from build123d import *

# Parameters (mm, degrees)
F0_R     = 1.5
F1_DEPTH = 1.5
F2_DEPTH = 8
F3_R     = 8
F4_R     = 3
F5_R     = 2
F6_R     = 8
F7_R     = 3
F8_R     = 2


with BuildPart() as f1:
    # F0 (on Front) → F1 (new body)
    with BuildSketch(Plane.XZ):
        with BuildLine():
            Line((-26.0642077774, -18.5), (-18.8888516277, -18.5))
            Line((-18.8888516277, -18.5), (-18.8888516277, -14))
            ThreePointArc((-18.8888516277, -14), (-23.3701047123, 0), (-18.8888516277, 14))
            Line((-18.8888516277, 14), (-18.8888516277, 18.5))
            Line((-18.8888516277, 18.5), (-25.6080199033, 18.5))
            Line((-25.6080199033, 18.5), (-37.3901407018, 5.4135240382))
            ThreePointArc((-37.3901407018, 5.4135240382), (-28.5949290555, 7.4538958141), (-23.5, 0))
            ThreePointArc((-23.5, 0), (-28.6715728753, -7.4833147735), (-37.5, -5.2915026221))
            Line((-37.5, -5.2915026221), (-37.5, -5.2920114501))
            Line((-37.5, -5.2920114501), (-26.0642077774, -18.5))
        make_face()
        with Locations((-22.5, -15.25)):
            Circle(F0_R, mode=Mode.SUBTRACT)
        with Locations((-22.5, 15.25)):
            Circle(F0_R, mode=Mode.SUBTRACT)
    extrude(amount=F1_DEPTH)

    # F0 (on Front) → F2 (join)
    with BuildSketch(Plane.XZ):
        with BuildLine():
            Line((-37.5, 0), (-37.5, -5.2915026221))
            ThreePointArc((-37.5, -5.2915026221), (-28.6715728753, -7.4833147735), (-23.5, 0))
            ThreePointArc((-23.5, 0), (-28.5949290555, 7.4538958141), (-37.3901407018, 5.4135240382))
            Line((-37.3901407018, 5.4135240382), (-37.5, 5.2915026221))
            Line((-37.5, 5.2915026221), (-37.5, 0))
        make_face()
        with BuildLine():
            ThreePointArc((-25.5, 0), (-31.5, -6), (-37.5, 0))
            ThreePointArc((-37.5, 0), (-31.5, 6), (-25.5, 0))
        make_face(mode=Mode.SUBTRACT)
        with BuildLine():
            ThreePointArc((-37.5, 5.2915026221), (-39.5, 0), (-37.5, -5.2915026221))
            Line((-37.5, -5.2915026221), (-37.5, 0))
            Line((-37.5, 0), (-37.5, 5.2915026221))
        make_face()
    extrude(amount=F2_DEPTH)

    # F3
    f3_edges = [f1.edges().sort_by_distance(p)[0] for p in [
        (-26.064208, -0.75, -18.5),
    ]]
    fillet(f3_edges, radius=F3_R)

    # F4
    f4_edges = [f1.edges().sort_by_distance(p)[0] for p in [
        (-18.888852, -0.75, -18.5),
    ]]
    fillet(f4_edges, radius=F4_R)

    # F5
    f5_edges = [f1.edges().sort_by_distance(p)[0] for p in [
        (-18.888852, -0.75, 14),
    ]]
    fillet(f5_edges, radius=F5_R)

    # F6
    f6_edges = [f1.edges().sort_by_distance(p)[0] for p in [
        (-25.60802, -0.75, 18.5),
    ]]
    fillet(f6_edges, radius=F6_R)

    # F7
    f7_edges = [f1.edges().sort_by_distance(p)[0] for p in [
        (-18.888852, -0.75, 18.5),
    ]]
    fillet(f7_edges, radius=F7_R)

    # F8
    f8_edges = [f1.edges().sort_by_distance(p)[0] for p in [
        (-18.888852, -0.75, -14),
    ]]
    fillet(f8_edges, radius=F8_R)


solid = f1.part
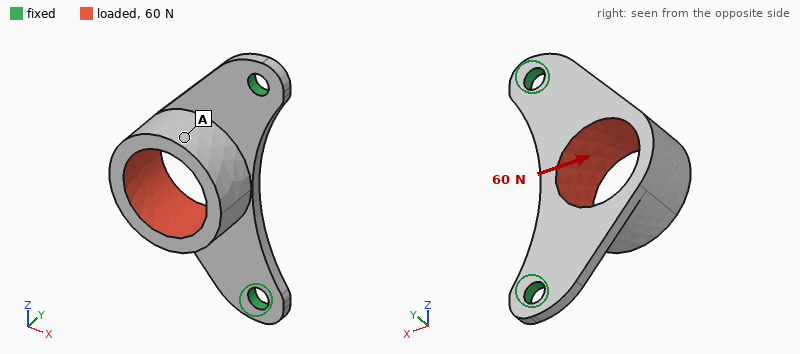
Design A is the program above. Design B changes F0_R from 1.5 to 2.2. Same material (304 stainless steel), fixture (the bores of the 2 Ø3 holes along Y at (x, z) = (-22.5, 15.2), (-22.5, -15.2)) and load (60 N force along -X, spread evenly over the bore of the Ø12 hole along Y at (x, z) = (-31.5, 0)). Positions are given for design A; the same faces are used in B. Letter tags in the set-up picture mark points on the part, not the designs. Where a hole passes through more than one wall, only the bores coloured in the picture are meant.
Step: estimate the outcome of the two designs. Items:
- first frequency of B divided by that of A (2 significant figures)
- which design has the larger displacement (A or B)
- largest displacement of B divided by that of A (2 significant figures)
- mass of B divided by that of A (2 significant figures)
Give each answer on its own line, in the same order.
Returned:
1.1
A
0.85
0.98
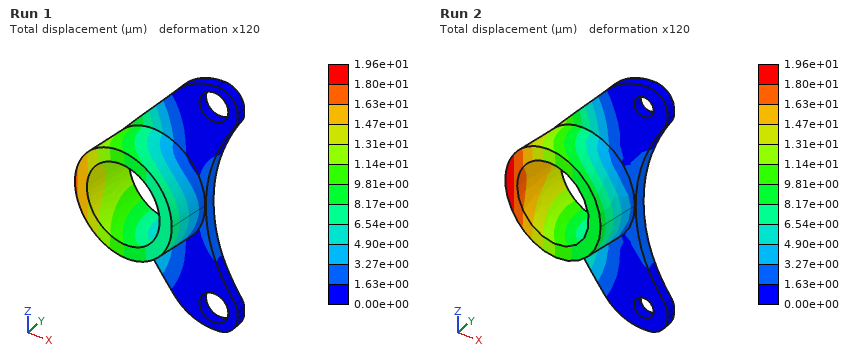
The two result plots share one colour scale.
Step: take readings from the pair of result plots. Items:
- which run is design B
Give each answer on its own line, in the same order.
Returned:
Run 1
